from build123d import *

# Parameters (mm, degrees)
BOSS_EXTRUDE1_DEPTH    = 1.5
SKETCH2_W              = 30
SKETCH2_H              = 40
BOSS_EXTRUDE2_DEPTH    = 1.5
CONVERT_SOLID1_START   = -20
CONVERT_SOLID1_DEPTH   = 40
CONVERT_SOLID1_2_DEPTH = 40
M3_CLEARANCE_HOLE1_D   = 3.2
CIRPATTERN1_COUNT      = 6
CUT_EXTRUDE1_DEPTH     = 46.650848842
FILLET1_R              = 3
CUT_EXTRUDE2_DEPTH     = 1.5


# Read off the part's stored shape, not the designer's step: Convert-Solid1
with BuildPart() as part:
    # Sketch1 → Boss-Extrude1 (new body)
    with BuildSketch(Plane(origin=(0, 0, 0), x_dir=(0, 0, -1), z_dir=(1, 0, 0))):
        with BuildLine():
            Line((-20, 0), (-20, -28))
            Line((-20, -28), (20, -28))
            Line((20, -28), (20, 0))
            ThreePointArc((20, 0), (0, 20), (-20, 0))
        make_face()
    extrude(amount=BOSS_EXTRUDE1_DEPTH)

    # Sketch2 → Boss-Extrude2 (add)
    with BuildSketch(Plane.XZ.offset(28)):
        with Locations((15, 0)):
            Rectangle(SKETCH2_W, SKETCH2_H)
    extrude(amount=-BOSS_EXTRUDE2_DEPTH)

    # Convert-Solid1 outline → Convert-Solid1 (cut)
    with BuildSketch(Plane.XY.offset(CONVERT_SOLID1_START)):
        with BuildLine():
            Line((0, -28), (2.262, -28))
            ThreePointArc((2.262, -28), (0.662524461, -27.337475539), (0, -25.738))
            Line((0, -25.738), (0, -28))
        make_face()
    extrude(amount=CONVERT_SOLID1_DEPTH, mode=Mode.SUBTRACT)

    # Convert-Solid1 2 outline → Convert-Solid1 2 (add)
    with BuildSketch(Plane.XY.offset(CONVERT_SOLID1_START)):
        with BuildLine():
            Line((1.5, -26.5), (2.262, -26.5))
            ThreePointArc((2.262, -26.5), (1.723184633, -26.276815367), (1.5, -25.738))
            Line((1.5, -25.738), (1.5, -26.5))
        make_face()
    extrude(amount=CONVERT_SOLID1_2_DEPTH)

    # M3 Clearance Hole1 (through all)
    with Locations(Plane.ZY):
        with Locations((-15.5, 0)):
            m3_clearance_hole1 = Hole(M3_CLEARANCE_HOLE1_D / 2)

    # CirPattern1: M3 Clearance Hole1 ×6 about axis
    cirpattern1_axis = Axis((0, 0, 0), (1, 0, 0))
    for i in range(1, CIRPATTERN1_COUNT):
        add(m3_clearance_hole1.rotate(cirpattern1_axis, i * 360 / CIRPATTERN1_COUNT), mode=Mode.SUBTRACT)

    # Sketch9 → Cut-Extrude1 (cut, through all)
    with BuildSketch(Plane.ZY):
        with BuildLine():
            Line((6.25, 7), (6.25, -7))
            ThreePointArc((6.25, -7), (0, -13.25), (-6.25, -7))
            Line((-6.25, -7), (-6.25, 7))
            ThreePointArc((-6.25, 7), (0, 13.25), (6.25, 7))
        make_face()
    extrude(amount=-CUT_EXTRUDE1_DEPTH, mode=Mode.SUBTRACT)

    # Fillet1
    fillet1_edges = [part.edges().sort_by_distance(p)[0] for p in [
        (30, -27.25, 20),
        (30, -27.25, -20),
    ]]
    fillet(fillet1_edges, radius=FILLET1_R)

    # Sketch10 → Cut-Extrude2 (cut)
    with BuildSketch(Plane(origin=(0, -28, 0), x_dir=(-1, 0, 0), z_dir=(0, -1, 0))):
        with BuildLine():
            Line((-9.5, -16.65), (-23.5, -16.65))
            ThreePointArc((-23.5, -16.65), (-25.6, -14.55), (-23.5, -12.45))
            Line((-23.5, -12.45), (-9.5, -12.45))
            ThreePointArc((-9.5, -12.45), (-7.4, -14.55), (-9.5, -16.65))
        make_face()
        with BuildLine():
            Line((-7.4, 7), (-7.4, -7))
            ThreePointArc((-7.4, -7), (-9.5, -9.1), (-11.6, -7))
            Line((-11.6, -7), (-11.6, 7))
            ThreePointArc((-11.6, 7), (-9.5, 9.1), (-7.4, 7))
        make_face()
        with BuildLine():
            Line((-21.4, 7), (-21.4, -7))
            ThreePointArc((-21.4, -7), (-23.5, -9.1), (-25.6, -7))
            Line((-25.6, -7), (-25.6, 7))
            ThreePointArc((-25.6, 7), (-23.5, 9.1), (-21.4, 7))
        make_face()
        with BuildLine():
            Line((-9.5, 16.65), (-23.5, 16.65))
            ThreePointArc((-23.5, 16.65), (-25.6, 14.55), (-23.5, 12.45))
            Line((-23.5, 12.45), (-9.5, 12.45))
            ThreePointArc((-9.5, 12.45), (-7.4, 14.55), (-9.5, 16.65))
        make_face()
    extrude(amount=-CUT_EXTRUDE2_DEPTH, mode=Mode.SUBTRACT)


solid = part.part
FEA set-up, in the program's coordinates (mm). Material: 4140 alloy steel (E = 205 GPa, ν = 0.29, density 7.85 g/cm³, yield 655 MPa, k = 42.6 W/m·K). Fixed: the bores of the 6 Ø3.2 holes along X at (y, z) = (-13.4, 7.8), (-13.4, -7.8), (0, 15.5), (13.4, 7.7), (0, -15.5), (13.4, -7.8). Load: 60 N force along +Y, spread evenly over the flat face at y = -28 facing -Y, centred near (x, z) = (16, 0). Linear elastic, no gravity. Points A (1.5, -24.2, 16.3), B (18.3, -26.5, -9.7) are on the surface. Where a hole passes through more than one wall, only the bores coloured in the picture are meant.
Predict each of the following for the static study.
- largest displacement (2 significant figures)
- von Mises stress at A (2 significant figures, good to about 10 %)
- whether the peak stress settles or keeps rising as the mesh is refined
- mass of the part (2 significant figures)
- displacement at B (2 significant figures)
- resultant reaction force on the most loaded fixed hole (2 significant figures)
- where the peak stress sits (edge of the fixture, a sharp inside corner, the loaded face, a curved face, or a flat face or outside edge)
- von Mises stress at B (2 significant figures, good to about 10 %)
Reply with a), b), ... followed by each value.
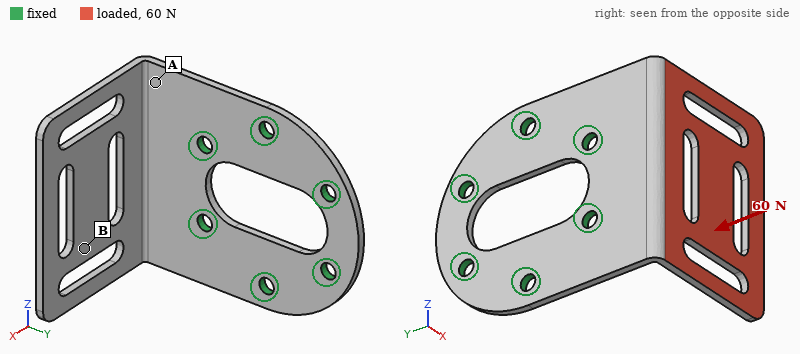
a) 0.31 mm
b) 63 MPa
c) keeps rising
d) 26 g
e) 0.16 mm
f) 26 N
g) a sharp inside corner
h) 15 MPa
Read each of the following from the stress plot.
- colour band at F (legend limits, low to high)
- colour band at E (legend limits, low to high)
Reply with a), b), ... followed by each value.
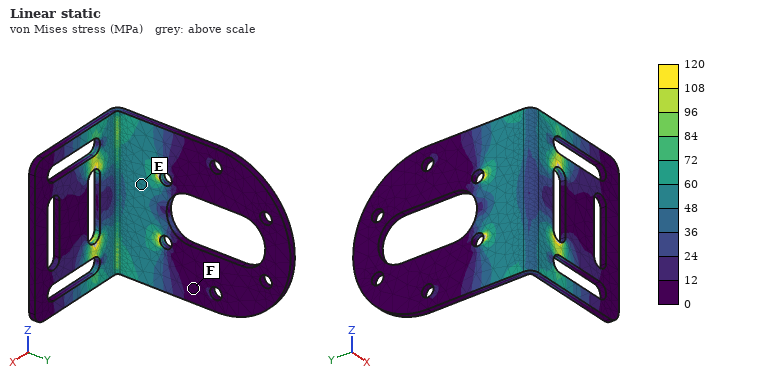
a) 0 to 12 MPa
b) 48 to 60 MPa
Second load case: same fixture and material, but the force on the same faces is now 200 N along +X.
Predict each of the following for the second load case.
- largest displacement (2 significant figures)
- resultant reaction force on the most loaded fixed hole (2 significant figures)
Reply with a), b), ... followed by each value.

a) 0.31 mm
b) 120 N
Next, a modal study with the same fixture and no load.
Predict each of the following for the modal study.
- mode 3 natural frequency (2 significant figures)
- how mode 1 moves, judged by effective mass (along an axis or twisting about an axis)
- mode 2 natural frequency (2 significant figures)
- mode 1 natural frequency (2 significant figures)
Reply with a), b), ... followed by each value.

a) 2700 Hz
b) along Y
c) 1700 Hz
d) 870 Hz
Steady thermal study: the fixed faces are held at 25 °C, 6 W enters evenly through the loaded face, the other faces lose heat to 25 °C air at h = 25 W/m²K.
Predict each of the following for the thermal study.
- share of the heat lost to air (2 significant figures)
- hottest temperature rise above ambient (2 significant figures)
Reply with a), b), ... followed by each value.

a) 36 %
b) 75 K
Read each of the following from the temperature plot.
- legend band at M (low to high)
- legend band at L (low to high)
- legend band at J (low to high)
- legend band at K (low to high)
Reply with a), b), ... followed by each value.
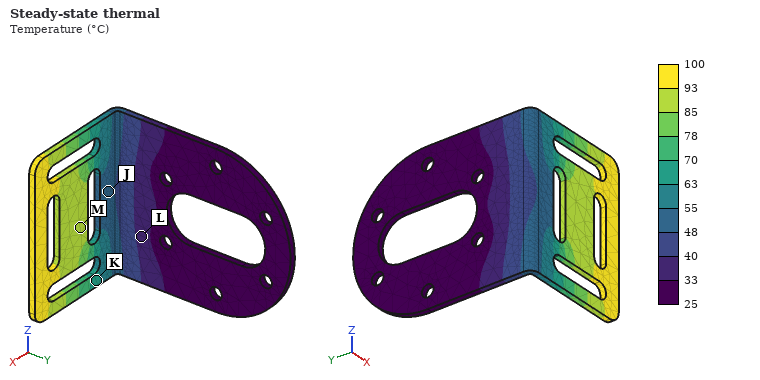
a) 85 to 93 °C
b) 33 to 40 °C
c) 48 to 55 °C
d) 63 to 70 °C
